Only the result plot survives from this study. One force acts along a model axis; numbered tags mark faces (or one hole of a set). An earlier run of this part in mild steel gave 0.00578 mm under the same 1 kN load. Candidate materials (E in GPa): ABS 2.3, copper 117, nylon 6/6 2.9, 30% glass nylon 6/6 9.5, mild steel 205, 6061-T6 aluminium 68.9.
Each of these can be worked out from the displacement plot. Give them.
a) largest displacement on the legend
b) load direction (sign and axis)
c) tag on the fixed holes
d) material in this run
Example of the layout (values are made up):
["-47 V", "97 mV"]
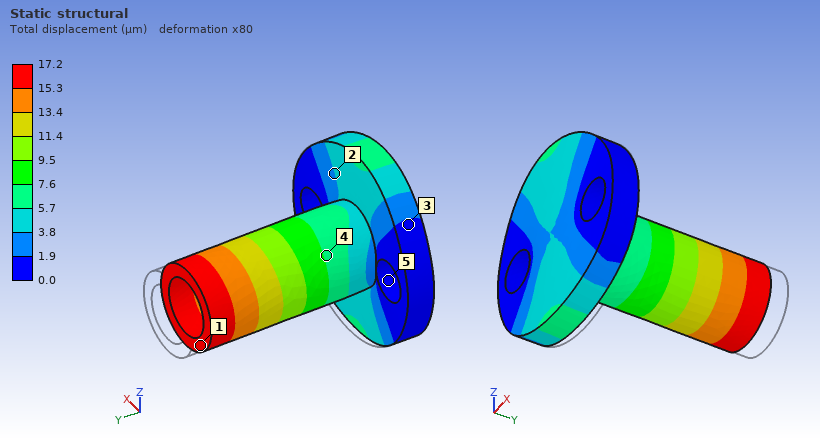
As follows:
["17.2 µm", "-Y", "5", "6061-T6 aluminium"]
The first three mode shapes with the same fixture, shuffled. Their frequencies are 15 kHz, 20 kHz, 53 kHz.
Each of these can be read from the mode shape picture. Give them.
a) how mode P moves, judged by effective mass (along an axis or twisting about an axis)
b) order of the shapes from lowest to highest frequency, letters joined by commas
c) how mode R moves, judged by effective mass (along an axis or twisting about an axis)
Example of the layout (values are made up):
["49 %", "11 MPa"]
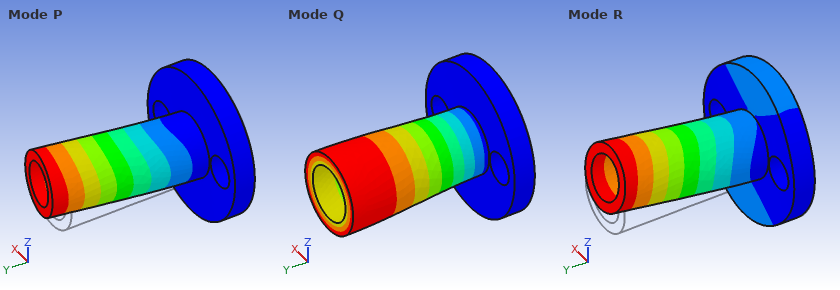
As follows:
["along X", "R, P, Q", "along Z"]
